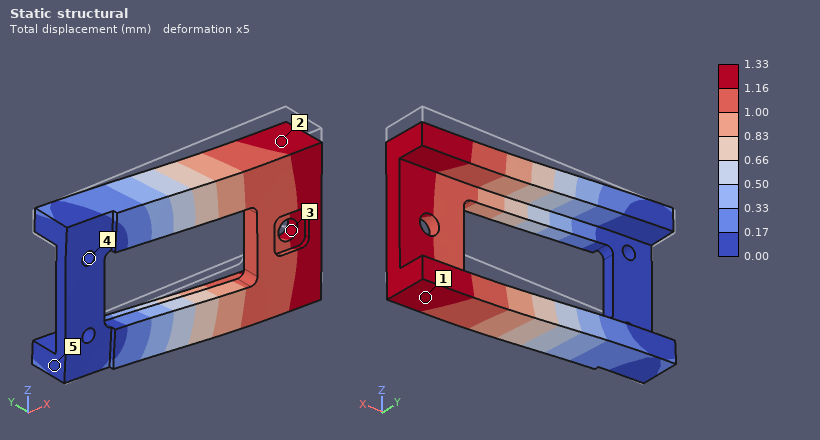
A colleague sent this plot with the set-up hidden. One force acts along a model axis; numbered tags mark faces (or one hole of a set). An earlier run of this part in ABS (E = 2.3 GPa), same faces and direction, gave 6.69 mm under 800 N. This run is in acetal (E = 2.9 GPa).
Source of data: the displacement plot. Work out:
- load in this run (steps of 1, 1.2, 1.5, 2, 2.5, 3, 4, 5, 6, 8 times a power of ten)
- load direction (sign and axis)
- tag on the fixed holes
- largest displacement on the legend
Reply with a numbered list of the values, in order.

1. 200 N
2. -Z
3. 4
4. 1.33 mm
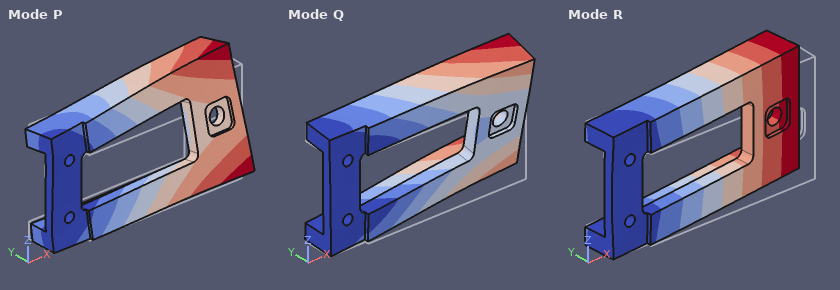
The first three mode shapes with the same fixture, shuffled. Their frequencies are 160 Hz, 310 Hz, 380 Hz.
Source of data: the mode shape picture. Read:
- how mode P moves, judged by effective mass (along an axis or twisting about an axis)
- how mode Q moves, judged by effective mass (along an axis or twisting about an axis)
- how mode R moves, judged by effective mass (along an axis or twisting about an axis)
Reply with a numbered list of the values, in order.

1. along Z
2. along Z
3. along Y
